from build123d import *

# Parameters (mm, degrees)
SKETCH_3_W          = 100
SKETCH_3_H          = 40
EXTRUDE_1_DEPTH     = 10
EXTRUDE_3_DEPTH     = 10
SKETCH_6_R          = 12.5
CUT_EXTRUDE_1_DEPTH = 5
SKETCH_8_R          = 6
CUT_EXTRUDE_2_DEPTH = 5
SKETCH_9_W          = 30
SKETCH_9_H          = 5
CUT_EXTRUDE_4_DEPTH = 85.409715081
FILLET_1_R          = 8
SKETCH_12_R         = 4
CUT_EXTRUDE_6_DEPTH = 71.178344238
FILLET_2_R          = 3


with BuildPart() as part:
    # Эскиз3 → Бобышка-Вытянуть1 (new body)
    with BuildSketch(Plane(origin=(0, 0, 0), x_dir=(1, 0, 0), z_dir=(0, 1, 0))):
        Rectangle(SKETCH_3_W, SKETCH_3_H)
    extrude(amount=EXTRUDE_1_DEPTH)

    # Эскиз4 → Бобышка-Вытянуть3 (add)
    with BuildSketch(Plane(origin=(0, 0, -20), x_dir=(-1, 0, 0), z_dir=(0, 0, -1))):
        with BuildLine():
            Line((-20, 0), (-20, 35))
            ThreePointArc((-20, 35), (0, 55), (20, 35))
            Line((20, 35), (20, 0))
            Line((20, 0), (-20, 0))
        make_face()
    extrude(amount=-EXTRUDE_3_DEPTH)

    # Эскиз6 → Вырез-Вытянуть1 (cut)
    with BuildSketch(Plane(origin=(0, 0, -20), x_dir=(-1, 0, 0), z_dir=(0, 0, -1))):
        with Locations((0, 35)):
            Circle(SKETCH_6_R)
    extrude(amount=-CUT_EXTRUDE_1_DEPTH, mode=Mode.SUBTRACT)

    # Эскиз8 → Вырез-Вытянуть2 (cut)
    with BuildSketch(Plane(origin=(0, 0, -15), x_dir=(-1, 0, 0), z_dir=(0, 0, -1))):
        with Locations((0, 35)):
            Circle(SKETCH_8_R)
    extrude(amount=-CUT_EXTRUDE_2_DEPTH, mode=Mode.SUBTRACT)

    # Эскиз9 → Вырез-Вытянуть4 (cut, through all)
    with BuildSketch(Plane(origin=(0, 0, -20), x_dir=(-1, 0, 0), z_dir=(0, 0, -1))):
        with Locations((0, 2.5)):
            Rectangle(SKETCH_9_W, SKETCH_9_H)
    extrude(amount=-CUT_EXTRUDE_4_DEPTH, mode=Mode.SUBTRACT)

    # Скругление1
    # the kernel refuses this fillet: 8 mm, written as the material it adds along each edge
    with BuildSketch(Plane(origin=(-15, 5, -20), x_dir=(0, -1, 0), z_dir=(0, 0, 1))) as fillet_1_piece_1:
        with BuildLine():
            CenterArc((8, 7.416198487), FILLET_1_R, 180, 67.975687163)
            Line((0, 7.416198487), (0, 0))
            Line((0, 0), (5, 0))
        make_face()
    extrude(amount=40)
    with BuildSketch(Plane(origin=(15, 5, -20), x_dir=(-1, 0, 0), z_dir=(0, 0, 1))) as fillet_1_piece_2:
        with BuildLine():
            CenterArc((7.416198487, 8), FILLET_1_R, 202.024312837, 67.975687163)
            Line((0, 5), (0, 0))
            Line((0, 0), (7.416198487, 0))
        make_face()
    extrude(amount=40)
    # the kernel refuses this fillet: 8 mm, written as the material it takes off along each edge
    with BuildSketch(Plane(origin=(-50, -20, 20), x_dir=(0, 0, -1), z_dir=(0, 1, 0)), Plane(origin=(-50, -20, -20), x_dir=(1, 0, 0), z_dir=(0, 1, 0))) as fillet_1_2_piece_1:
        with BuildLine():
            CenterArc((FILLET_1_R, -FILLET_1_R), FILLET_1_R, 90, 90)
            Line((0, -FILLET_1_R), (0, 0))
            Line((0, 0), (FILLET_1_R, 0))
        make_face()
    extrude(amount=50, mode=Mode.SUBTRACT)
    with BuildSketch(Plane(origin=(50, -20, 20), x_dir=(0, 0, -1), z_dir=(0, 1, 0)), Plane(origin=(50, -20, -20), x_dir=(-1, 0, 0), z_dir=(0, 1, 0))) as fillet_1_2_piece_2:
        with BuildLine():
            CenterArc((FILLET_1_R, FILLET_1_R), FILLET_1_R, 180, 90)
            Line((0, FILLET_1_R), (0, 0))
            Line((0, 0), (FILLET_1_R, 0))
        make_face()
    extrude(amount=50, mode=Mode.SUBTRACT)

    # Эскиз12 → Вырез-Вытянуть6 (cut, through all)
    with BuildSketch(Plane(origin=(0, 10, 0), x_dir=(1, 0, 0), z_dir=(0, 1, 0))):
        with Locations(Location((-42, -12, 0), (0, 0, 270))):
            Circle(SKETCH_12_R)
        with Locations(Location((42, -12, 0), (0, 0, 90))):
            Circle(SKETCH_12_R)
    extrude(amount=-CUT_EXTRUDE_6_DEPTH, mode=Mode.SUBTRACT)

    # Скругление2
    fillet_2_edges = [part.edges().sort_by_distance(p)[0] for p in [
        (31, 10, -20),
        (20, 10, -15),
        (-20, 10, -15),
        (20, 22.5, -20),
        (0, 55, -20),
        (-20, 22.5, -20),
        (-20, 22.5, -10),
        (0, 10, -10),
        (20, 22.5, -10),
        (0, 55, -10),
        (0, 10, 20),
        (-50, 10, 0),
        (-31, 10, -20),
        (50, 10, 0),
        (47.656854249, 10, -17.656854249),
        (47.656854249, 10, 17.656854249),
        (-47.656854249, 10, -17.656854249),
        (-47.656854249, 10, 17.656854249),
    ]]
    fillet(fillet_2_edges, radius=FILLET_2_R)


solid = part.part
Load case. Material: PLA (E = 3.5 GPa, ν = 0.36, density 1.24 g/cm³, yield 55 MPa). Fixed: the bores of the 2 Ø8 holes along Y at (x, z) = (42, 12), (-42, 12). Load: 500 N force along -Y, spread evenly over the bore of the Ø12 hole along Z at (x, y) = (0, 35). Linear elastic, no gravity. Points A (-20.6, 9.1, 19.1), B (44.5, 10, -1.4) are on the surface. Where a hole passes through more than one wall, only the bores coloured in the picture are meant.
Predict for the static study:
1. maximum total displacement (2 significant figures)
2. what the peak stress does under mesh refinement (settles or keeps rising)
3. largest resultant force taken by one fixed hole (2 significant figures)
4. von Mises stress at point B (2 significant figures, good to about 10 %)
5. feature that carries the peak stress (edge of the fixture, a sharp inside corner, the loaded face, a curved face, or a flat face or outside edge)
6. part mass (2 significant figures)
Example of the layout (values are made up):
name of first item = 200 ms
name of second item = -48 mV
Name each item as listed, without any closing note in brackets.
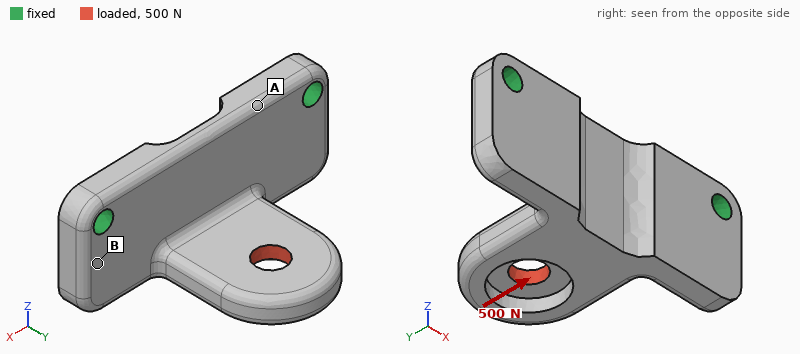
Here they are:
maximum total displacement = 0.60 mm
what the peak stress does under mesh refinement = keeps rising
largest resultant force taken by one fixed hole = 270 N
von Mises stress at point B = 7.4 MPa
feature that carries the peak stress = edge of the fixture
part mass = 57 g
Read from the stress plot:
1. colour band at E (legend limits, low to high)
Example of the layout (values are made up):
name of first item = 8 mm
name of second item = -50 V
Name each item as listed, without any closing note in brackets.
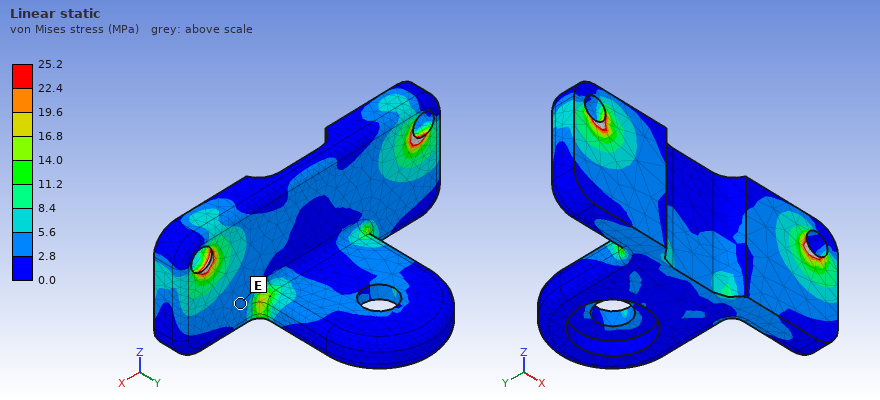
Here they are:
colour band at E = 2.8 to 5.6 MPa
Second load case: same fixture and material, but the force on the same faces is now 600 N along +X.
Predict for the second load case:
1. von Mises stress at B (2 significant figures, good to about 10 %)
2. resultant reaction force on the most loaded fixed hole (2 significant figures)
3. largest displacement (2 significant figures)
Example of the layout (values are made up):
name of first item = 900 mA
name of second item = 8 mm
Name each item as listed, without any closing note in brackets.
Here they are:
von Mises stress at B = 5.0 MPa
resultant reaction force on the most loaded fixed hole = 430 N
largest displacement = 0.58 mm
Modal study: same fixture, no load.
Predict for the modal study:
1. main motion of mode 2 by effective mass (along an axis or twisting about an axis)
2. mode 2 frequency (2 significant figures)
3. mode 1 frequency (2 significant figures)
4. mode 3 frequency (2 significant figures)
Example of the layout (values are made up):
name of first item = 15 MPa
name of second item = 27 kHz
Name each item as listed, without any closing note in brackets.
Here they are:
main motion of mode 2 by effective mass = along Y
mode 2 frequency = 1400 Hz
mode 1 frequency = 740 Hz
mode 3 frequency = 1500 Hz
